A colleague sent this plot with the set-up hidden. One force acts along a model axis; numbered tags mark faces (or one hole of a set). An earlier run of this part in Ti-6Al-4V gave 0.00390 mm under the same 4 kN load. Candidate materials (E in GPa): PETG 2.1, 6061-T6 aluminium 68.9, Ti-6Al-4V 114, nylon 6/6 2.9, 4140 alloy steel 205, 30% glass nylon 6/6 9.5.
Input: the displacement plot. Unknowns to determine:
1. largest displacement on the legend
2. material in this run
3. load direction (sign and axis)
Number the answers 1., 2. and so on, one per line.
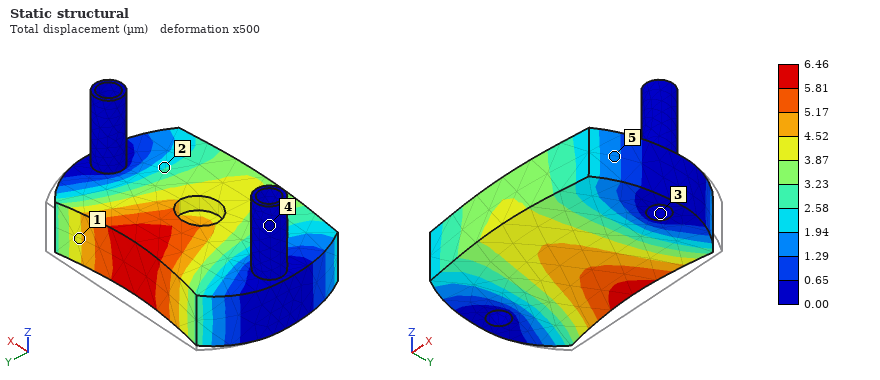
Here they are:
1. 6.46 µm
2. 6061-T6 aluminium
3. -Y
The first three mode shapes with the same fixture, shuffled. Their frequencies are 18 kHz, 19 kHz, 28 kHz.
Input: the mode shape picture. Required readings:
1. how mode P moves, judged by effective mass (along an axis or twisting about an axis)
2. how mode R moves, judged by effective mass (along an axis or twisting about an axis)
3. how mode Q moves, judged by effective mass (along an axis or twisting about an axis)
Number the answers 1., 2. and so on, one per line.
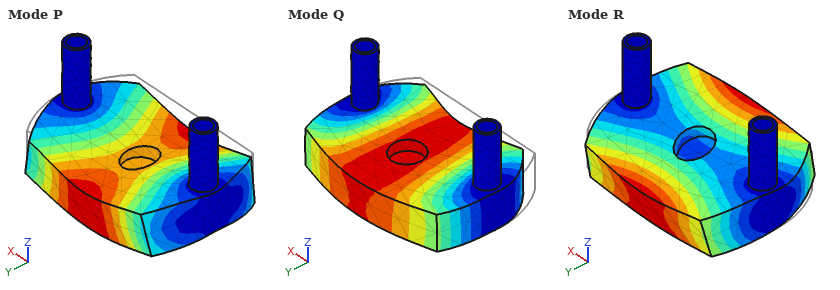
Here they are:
1. along Z
2. twisting about X
3. along Y
